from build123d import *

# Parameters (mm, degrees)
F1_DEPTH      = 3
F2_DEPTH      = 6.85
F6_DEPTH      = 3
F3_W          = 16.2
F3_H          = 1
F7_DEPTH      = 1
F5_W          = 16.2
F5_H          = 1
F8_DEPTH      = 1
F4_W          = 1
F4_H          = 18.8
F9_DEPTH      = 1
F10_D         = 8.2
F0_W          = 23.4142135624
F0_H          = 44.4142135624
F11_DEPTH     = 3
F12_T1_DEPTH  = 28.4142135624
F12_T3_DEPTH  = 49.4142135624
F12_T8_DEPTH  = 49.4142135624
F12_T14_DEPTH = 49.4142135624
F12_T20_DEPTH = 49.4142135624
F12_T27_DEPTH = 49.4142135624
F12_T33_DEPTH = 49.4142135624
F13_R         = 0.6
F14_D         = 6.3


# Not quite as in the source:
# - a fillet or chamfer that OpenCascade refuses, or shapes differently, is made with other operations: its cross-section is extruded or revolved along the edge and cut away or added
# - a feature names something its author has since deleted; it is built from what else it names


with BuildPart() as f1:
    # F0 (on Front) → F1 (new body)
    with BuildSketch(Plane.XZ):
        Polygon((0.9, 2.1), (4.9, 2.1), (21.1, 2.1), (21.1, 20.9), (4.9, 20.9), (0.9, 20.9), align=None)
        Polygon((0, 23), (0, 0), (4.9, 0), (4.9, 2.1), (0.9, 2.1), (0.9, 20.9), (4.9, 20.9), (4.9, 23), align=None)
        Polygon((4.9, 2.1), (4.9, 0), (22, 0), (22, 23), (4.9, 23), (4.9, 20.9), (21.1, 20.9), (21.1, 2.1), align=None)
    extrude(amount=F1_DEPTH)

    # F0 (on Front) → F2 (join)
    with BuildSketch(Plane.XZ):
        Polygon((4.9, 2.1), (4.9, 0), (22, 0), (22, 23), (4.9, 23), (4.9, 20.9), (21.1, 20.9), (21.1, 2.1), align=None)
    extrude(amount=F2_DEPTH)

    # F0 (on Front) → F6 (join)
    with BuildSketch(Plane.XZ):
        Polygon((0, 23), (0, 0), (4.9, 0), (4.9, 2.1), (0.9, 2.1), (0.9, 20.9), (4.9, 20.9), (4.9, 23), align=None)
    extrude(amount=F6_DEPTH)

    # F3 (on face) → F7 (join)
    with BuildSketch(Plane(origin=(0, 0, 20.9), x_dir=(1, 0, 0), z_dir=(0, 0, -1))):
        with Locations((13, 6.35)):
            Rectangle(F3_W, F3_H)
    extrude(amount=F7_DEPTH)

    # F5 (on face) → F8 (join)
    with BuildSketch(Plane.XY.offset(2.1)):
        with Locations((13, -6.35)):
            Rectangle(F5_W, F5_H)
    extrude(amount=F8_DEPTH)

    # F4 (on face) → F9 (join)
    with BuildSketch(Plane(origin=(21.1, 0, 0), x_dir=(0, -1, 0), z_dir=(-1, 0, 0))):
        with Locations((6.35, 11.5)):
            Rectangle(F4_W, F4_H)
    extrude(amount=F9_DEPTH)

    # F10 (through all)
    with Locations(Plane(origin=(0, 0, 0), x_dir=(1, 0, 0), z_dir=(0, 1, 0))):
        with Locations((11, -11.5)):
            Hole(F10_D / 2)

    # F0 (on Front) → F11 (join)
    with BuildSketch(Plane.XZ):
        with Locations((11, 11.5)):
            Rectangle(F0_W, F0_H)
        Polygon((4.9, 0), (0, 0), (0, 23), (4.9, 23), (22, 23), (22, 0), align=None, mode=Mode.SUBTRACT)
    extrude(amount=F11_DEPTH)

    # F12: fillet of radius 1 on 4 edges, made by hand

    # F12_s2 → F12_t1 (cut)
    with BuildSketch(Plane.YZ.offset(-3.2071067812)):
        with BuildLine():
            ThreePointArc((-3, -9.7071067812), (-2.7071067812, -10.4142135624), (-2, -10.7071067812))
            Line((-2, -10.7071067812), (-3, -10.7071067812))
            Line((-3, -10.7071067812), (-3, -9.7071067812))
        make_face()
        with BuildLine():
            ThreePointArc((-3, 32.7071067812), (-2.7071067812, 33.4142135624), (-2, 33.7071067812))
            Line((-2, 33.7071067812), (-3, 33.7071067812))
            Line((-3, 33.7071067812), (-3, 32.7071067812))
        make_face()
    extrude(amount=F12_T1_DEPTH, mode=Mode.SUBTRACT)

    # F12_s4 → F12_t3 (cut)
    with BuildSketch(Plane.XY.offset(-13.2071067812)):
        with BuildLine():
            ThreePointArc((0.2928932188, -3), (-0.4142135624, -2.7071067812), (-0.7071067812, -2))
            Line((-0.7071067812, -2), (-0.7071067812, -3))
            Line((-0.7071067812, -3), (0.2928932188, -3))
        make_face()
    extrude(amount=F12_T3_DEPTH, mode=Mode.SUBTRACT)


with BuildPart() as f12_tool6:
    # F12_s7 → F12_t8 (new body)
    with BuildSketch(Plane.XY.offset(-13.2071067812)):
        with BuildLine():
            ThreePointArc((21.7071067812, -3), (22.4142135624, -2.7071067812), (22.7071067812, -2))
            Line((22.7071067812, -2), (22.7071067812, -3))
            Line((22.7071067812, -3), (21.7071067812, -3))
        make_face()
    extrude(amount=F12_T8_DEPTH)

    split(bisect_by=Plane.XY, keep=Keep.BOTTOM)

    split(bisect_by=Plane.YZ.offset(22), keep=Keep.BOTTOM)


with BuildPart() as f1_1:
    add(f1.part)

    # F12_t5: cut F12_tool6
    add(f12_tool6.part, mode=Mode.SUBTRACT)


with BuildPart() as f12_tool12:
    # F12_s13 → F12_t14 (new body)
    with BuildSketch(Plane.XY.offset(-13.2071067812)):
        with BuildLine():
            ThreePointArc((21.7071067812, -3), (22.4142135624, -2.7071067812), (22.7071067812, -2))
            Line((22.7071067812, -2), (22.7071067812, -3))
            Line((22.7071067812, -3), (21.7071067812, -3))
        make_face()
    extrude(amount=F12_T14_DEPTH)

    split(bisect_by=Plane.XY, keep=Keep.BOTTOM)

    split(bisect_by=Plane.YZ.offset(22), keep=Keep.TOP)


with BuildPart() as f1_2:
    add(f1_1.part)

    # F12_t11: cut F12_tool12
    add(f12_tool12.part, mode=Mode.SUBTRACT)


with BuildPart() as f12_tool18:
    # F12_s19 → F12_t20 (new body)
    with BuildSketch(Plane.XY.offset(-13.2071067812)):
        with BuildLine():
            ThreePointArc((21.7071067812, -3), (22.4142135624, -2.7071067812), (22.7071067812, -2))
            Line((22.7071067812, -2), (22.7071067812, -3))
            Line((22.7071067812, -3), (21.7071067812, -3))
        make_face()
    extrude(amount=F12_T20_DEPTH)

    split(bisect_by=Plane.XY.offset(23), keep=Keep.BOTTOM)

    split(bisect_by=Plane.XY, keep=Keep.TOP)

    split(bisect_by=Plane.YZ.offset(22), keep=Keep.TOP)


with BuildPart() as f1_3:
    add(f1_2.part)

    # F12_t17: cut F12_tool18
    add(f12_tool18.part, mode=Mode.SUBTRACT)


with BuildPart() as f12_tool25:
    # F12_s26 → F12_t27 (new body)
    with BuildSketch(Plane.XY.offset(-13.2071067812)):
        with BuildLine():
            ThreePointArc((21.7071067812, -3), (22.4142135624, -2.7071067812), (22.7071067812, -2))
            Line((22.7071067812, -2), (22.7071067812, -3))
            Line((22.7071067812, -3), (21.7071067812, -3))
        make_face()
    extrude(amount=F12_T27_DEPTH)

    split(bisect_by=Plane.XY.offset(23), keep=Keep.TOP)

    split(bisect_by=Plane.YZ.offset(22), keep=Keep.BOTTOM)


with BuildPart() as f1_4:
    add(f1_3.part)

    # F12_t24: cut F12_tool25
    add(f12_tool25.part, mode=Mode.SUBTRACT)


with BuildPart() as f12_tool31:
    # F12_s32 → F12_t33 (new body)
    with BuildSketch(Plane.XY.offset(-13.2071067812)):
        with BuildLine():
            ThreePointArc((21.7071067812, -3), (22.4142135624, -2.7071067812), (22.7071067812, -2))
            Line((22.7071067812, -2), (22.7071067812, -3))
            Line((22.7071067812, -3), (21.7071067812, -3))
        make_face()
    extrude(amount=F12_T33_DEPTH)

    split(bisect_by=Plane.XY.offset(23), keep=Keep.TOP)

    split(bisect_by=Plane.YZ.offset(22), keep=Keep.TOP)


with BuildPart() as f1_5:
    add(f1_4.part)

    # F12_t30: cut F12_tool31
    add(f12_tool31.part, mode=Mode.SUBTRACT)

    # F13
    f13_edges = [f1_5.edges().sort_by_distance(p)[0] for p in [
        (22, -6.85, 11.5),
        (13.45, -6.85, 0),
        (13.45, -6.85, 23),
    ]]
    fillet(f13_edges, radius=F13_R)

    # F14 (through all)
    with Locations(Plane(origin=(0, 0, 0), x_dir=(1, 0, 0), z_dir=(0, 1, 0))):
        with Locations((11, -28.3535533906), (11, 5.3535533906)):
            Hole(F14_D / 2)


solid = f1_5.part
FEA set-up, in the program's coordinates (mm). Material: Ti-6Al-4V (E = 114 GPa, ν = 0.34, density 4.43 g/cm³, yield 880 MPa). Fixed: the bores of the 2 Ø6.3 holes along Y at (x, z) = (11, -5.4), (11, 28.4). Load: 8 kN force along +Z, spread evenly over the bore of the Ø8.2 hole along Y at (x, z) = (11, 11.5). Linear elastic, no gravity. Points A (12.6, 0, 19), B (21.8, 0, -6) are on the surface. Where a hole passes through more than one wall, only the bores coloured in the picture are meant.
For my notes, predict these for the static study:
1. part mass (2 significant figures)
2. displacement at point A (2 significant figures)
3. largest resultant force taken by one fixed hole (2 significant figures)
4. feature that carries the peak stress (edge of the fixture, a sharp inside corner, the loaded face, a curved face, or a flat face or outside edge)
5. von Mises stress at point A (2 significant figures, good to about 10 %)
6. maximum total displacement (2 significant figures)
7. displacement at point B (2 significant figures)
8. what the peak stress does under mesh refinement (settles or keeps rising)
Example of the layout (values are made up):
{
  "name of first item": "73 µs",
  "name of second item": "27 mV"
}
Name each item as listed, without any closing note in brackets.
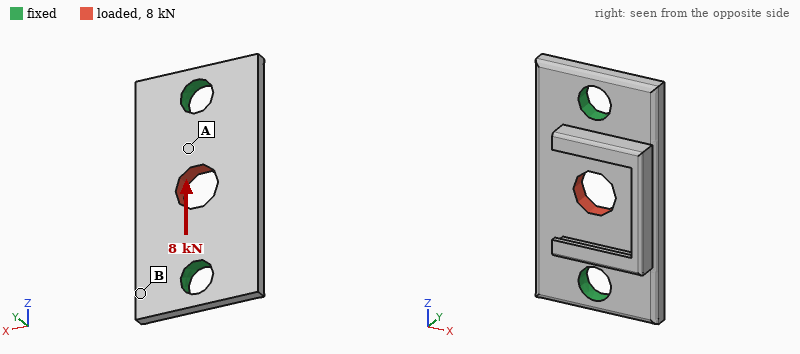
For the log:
{
  "part mass": "14 g",
  "displacement at point A": "7.0 µm",
  "largest resultant force taken by one fixed hole": "4.0 kN",
  "feature that carries the peak stress": "a sharp inside corner",
  "von Mises stress at point A": "120 MPa",
  "maximum total displacement": "13 µm",
  "displacement at point B": "5.7 µm",
  "what the peak stress does under mesh refinement": "keeps rising"
}
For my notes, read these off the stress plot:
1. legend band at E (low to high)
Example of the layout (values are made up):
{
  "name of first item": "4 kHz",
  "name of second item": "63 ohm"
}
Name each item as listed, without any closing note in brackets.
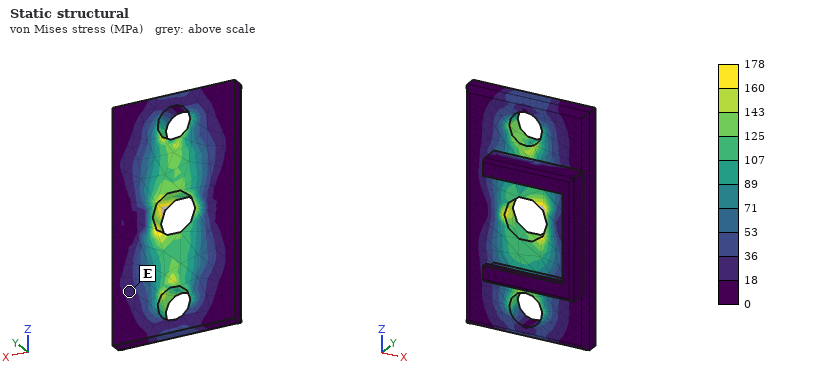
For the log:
{
  "legend band at E": "18 to 36 MPa"
}
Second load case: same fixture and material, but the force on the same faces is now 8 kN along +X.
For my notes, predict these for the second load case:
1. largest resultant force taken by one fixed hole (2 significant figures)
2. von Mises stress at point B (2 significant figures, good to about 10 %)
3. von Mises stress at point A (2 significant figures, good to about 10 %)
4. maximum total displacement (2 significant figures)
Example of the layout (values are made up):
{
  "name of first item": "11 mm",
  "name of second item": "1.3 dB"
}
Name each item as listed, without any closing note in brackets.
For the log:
{
  "largest resultant force taken by one fixed hole": "4.0 kN",
  "von Mises stress at point B": "21 MPa",
  "von Mises stress at point A": "130 MPa",
  "maximum total displacement": "31 µm"
}
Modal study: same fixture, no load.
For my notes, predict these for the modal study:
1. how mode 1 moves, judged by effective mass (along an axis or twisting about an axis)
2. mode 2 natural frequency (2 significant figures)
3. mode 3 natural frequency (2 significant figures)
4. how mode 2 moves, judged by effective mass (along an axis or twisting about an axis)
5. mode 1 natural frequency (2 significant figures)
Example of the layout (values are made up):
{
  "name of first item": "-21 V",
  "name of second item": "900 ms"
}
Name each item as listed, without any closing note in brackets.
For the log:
{
  "how mode 1 moves, judged by effective mass": "twisting about Z",
  "mode 2 natural frequency": "16 kHz",
  "mode 3 natural frequency": "25 kHz",
  "how mode 2 moves, judged by effective mass": "along Y",
  "mode 1 natural frequency": "14 kHz"
}
